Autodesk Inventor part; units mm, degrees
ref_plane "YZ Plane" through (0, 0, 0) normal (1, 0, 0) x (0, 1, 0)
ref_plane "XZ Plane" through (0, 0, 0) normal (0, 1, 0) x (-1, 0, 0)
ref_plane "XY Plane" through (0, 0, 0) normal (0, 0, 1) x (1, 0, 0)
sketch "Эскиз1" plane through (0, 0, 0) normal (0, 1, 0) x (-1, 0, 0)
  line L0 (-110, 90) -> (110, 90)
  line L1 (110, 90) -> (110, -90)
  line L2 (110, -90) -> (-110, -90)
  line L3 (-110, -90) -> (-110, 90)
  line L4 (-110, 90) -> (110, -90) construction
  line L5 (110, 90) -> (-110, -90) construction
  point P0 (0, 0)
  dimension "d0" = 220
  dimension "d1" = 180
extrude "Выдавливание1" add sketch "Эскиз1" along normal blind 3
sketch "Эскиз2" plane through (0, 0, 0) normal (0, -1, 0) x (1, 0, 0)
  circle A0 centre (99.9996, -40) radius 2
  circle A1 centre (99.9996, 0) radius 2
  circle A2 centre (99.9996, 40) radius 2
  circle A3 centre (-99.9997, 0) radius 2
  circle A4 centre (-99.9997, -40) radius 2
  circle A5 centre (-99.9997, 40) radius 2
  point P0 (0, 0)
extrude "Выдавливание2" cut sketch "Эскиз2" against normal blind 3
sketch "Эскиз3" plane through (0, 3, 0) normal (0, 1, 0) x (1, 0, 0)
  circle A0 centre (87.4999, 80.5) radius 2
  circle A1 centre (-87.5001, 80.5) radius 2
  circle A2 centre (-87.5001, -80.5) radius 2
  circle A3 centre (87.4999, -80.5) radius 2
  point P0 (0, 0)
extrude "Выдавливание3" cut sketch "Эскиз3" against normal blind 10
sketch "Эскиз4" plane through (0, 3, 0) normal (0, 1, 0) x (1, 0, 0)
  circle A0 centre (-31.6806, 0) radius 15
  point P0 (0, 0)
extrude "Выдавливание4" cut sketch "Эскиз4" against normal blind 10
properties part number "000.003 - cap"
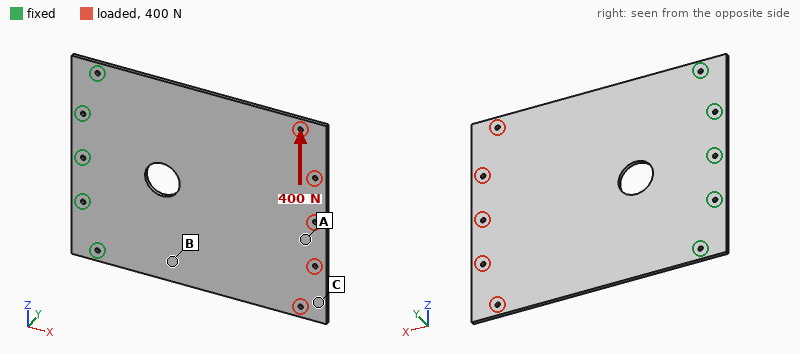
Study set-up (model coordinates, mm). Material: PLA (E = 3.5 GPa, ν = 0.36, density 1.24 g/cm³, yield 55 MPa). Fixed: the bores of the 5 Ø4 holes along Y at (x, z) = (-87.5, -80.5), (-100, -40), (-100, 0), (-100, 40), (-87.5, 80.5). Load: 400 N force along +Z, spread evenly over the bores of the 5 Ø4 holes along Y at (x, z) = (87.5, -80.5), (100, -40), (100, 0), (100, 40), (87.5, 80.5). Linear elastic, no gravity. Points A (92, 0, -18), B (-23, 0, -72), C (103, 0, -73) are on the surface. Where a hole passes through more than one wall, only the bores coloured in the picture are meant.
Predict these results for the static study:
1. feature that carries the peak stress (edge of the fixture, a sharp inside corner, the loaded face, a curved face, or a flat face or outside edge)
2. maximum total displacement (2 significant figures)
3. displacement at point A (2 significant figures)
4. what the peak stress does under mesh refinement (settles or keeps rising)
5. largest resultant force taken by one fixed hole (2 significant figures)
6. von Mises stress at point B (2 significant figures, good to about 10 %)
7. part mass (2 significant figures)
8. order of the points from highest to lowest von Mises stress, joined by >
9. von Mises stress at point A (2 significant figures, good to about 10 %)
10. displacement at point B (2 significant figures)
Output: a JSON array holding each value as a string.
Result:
["edge of the fixture", "0.38 mm", "0.32 mm", "keeps rising", "410 N", "2.5 MPa", "140 g", "B > A > C", "1.4 MPa", "0.12 mm"]
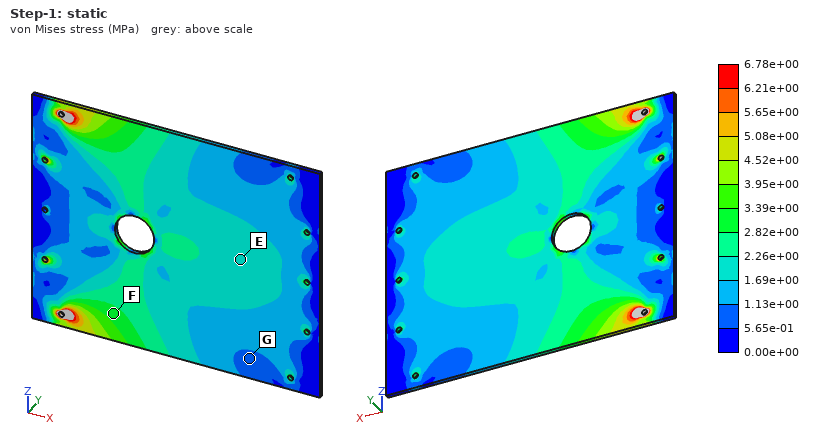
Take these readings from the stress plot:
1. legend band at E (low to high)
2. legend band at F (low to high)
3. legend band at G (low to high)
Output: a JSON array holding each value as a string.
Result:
["1.69e+00 to 2.26e+00 MPa", "2.82e+00 to 3.39e+00 MPa", "5.65e-01 to 1.13e+00 MPa"]
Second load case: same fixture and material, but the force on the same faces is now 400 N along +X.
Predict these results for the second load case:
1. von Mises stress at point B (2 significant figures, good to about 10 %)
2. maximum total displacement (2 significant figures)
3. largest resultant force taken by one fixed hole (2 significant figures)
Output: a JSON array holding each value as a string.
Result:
["0.79 MPa", "50 µm", "93 N"]
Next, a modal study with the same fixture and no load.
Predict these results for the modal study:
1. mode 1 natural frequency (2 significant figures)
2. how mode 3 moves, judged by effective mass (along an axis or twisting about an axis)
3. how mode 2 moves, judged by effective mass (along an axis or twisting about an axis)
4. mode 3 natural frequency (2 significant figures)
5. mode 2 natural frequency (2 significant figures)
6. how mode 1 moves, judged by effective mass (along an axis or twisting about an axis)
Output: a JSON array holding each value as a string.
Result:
["19 Hz", "along Y", "twisting about X", "120 Hz", "54 Hz", "along Y"]
